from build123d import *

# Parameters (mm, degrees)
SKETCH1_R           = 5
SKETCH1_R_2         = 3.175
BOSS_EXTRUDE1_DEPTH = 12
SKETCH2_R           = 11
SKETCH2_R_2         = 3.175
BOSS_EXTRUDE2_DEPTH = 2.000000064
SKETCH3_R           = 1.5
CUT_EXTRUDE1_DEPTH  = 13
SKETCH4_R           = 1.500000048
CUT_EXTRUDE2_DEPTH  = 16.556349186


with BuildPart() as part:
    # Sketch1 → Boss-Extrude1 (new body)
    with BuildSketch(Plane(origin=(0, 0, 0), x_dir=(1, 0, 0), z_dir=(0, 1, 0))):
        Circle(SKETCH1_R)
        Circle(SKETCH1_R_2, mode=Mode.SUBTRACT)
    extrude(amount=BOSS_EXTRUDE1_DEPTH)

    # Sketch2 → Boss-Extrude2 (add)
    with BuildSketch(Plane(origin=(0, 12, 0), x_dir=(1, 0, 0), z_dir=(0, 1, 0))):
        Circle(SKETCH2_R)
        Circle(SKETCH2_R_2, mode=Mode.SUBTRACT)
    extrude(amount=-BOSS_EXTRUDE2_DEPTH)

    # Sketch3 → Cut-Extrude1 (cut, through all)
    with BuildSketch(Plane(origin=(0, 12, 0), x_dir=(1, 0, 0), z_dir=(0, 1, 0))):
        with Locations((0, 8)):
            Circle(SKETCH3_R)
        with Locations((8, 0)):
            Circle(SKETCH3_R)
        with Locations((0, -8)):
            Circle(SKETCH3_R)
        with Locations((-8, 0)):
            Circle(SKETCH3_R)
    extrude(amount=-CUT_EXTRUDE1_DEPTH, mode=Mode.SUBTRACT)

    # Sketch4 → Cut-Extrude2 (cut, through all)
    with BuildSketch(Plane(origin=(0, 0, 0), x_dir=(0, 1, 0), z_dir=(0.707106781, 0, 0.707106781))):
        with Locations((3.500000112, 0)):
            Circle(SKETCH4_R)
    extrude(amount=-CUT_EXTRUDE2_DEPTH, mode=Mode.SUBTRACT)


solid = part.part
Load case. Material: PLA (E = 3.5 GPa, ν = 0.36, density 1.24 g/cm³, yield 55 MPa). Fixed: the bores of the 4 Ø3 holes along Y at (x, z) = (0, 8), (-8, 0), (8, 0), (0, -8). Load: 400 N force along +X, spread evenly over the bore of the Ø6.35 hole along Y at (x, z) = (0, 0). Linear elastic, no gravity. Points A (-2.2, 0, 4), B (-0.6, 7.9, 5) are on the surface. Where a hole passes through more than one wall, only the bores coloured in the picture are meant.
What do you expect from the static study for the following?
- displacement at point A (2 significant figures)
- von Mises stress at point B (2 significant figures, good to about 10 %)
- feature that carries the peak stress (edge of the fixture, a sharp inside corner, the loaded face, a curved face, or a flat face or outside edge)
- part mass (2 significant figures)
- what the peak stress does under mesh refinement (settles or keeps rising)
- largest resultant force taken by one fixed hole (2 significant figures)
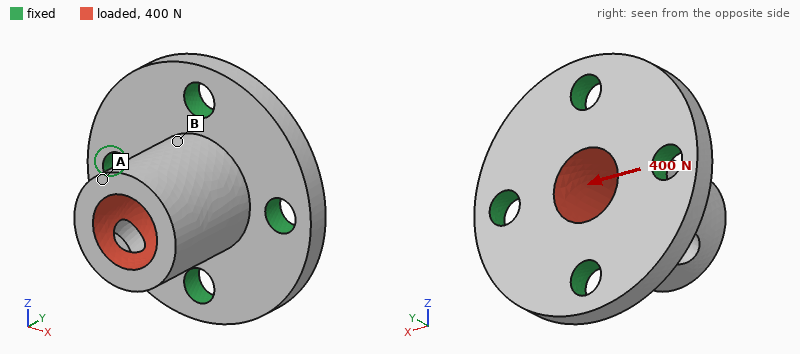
0.17 mm
10 MPa
edge of the fixture
1.4 g
keeps rising
200 N
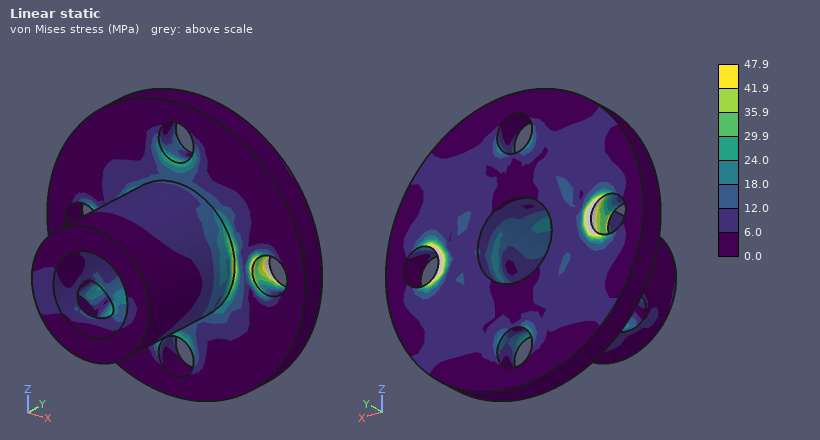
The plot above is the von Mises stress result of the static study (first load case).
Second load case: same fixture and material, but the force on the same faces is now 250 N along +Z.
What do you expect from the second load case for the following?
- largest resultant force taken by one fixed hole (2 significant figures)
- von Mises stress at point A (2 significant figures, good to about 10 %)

130 N
3.0 MPa
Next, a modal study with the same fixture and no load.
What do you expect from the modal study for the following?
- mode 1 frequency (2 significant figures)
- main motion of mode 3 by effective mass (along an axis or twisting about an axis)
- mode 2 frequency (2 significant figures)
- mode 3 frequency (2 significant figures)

10 kHz
along Y
10 kHz
18 kHz
